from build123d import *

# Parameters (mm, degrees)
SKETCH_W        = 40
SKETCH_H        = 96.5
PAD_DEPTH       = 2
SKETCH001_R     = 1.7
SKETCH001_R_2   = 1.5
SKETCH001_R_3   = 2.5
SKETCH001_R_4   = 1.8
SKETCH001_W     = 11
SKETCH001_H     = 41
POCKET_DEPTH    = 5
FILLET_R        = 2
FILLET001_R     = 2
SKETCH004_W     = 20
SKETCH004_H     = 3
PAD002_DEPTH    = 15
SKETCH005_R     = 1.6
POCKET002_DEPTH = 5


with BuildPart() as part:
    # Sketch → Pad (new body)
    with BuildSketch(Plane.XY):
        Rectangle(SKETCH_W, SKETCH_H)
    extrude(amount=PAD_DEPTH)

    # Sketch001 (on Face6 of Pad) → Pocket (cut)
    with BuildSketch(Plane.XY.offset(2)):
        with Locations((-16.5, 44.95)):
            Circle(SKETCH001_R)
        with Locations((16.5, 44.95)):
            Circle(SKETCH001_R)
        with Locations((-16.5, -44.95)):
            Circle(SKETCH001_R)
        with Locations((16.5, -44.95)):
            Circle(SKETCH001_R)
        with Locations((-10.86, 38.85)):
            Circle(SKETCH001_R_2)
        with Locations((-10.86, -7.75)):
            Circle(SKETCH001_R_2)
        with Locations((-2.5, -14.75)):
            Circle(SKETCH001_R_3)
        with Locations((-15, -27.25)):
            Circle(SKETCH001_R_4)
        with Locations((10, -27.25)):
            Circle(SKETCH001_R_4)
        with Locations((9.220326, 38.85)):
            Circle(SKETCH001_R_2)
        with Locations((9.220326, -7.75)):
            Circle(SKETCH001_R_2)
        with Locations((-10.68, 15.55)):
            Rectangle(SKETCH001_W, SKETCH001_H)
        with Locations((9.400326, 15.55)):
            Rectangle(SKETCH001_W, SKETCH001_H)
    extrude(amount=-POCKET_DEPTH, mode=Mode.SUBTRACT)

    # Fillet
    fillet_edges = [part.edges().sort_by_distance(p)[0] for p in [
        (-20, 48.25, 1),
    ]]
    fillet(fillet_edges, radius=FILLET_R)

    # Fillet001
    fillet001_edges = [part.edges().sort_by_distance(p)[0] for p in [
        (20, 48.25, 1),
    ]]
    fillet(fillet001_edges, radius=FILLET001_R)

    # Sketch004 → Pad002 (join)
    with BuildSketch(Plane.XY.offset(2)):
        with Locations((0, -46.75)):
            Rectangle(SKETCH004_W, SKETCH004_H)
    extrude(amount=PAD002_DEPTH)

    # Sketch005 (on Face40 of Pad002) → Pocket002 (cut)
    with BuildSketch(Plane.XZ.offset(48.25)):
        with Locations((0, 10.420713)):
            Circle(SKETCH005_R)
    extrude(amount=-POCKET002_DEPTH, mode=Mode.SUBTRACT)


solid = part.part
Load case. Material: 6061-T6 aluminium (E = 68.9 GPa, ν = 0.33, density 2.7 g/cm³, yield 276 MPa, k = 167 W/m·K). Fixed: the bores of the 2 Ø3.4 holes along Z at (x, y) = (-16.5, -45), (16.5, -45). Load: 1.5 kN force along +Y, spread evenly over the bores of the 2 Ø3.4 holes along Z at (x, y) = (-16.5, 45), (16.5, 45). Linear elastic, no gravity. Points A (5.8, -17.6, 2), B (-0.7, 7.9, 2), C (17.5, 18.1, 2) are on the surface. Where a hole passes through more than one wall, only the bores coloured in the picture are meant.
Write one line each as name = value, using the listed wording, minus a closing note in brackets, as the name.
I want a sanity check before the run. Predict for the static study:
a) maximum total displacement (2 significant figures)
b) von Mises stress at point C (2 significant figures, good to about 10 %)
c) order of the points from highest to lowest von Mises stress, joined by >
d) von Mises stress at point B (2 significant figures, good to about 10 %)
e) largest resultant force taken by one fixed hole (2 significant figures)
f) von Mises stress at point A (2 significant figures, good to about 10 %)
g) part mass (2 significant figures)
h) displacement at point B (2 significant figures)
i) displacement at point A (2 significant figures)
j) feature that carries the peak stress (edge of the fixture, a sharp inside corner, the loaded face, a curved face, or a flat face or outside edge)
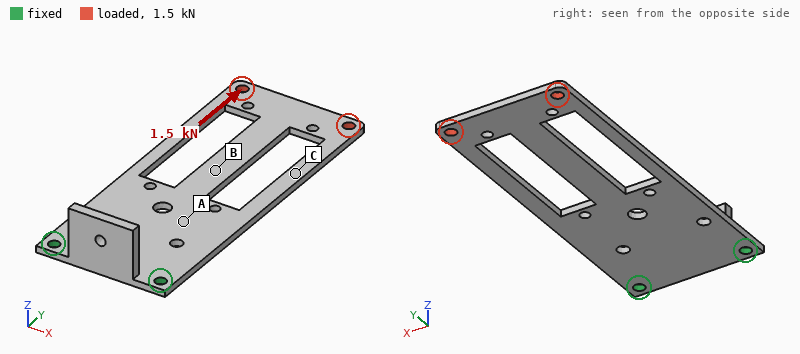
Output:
maximum total displacement = 66 µm
von Mises stress at point C = 48 MPa
order of the points from highest to lowest von Mises stress, joined by > = C > B > A
von Mises stress at point B = 31 MPa
largest resultant force taken by one fixed hole = 770 N
von Mises stress at point A = 14 MPa
part mass = 18 g
displacement at point B = 21 µm
displacement at point A = 11 µm
feature that carries the peak stress = the loaded face
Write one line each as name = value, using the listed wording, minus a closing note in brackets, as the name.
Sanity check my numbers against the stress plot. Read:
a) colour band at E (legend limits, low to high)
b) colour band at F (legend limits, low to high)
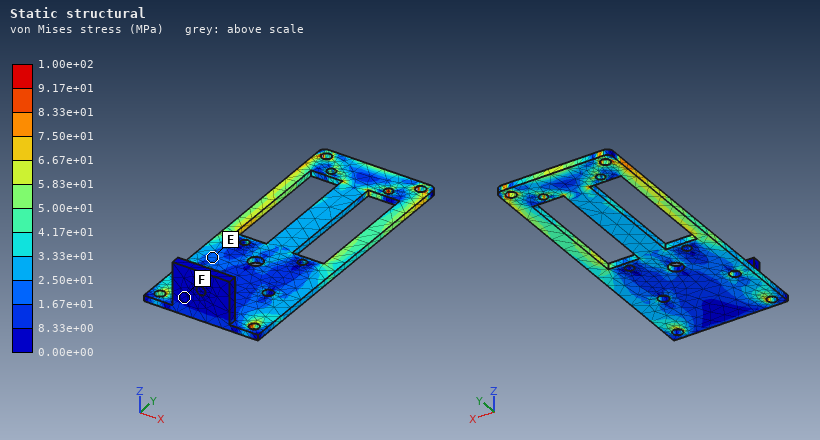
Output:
colour band at E = 1.67e+01 to 2.50e+01 MPa
colour band at F = 0.00e+00 to 8.33e+00 MPa
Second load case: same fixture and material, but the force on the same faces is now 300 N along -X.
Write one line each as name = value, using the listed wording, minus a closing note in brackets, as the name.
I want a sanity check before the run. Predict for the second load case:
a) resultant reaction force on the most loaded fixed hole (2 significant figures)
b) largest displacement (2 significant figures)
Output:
resultant reaction force on the most loaded fixed hole = 820 N
largest displacement = 0.40 mm
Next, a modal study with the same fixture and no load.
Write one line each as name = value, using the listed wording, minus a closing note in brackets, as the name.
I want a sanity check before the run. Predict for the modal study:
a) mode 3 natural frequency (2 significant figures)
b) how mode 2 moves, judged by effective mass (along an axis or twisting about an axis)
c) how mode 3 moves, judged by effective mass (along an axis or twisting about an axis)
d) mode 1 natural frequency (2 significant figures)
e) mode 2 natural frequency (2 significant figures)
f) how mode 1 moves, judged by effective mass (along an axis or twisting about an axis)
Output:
mode 3 natural frequency = 1100 Hz
how mode 2 moves, judged by effective mass = twisting about Y
how mode 3 moves, judged by effective mass = along Z
mode 1 natural frequency = 200 Hz
mode 2 natural frequency = 890 Hz
how mode 1 moves, judged by effective mass = along Z
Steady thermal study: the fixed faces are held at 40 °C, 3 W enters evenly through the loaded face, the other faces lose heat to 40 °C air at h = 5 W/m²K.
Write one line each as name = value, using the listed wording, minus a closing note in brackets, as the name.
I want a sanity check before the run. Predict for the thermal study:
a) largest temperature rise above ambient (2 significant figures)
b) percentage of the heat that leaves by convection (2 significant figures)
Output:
largest temperature rise above ambient = 34 K
percentage of the heat that leaves by convection = 15 %
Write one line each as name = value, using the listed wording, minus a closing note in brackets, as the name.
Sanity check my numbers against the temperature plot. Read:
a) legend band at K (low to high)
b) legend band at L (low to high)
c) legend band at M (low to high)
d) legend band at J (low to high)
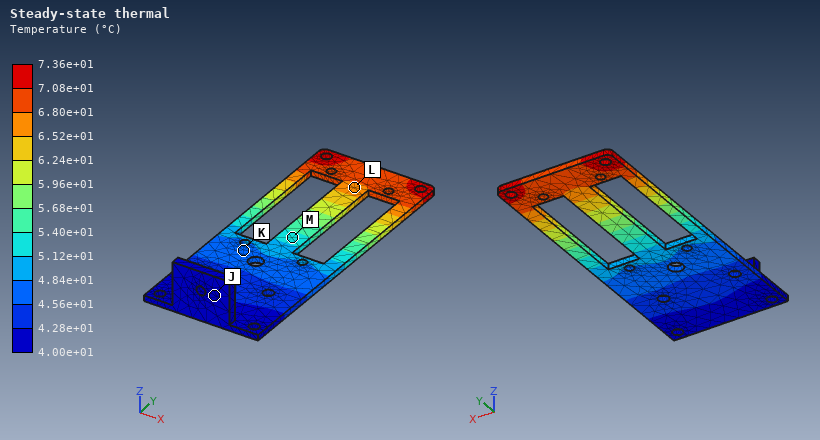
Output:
legend band at K = 4.56e+01 to 4.84e+01 °C
legend band at L = 6.52e+01 to 6.80e+01 °C
legend band at M = 5.12e+01 to 5.40e+01 °C
legend band at J = 4.00e+01 to 4.28e+01 °C
